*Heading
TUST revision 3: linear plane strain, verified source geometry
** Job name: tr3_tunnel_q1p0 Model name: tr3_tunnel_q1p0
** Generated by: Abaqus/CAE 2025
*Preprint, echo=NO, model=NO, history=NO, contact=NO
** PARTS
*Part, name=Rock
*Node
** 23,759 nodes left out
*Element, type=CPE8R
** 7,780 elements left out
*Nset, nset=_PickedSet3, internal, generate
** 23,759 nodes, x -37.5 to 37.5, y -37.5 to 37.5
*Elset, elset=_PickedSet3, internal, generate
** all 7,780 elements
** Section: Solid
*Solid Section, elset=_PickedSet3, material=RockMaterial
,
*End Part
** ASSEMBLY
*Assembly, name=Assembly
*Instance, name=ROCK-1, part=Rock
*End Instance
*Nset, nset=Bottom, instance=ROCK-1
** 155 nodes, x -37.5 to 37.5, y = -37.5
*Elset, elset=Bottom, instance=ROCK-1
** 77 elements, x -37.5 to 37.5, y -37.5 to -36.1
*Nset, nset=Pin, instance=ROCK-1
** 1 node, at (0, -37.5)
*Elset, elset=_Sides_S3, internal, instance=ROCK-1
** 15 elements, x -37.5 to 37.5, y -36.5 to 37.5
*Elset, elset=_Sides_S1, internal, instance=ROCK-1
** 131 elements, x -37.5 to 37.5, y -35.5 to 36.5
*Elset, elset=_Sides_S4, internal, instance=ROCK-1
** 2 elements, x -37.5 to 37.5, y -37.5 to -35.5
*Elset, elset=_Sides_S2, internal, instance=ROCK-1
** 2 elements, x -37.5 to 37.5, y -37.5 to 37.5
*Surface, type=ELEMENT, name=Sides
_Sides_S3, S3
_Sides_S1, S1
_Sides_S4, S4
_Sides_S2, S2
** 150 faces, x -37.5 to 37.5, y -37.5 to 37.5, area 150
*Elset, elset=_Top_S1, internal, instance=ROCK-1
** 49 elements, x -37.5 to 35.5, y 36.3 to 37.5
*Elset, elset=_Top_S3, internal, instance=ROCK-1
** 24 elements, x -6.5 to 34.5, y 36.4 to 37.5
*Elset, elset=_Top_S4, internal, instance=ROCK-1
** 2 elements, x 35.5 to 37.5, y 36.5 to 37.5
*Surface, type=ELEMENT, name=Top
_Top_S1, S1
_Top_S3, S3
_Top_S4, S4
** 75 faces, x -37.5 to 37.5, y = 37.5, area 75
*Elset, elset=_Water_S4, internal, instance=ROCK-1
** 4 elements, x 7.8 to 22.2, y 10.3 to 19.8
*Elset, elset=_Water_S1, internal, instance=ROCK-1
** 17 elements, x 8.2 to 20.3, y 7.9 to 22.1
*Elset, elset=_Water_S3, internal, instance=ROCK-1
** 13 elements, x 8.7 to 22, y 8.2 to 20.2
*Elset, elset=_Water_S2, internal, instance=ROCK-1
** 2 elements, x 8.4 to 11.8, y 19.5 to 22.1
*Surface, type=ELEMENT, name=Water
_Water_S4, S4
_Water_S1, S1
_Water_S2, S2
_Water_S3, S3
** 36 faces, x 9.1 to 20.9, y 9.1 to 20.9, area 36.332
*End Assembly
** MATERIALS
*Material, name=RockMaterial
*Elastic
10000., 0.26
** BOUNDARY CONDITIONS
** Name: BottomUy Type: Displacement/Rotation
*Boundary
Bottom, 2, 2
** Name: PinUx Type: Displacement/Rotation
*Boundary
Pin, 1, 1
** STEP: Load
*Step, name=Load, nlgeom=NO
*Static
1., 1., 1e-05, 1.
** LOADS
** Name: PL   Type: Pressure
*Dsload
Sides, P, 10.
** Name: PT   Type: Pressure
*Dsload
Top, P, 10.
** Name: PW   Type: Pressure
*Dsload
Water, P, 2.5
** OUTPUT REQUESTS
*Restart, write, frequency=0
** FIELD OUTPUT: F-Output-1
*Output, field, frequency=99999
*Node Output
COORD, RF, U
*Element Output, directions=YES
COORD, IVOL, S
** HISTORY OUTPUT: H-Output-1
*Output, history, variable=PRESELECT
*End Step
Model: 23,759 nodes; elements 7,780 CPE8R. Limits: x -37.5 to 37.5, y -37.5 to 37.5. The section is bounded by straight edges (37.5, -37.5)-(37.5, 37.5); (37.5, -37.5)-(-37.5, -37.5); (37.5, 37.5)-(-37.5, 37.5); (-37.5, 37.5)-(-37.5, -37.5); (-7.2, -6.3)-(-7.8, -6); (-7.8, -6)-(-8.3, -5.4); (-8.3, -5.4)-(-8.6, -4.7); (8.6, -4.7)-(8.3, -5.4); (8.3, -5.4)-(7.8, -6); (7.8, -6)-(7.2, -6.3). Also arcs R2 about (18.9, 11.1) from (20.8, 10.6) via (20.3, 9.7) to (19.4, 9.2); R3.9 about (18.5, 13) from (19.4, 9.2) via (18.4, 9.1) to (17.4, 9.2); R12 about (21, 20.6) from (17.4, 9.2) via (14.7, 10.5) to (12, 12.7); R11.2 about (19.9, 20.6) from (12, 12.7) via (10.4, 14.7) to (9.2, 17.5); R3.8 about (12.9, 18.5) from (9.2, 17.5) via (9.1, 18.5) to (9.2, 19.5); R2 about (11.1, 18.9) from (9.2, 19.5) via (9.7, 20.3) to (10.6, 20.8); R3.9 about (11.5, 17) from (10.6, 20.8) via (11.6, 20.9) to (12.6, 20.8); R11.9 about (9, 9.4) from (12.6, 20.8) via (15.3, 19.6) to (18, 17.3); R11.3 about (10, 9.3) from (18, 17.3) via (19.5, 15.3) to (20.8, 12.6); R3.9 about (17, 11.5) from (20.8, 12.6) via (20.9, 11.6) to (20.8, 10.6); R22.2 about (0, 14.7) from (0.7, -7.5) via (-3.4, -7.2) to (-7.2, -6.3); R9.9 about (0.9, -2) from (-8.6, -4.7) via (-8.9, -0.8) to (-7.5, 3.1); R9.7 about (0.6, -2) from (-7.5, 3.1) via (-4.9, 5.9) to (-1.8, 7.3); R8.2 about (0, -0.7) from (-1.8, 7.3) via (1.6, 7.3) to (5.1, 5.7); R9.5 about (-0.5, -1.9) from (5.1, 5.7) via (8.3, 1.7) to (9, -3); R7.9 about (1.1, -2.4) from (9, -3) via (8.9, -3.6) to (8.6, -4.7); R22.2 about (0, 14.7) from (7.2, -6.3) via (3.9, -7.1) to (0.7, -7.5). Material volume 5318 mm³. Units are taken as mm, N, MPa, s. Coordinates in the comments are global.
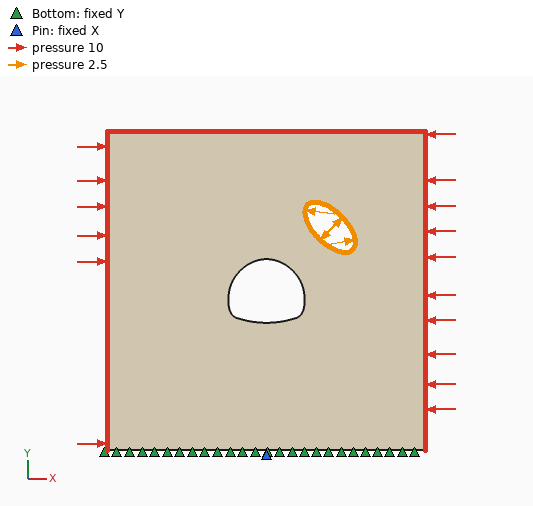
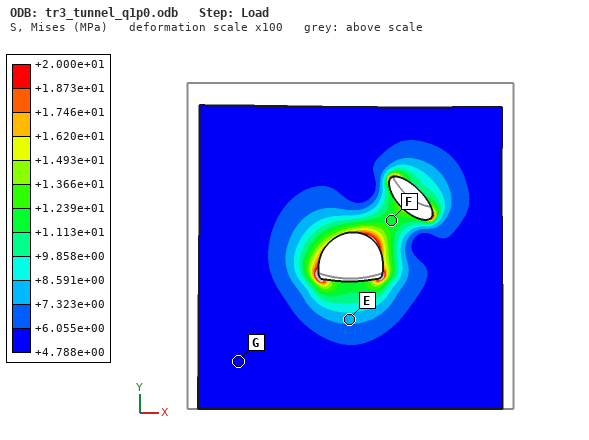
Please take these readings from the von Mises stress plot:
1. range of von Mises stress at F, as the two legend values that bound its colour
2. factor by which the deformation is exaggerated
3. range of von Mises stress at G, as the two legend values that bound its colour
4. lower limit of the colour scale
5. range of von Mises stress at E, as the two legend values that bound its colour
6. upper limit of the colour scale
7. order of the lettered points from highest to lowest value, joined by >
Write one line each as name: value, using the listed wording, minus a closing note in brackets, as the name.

range of von Mises stress at F, as the two legend values that bound its colour: +1.113e+01 to +1.239e+01 MPa
factor by which the deformation is exaggerated: 100
range of von Mises stress at G, as the two legend values that bound its colour: +4.788e+00 to +6.055e+00 MPa
lower limit of the colour scale: +4.788e+00 MPa
range of von Mises stress at E, as the two legend values that bound its colour: +7.323e+00 to +8.591e+00 MPa
upper limit of the colour scale: +2.000e+01 MPa
order of the lettered points from highest to lowest value, joined by >: F > E > G
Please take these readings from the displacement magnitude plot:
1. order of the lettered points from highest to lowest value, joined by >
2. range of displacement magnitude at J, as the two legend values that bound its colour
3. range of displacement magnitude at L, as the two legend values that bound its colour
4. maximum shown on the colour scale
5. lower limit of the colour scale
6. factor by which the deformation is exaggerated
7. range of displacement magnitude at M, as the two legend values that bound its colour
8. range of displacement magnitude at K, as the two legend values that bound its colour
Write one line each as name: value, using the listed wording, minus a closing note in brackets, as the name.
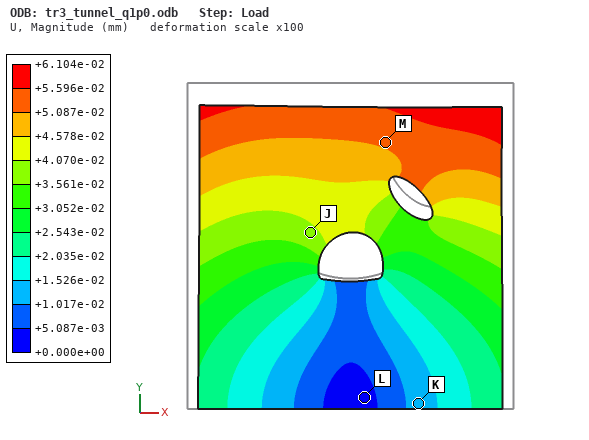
order of the lettered points from highest to lowest value, joined by >: M > J > K > L
range of displacement magnitude at J, as the two legend values that bound its colour: +3.561e-02 to +4.070e-02 mm
range of displacement magnitude at L, as the two legend values that bound its colour: +0.000e+00 to +5.087e-03 mm
maximum shown on the colour scale: +6.104e-02 mm
lower limit of the colour scale: +0.000e+00 mm
factor by which the deformation is exaggerated: 100
range of displacement magnitude at M, as the two legend values that bound its colour: +5.087e-02 to +5.596e-02 mm
range of displacement magnitude at K, as the two legend values that bound its colour: +1.017e-02 to +1.526e-02 mm
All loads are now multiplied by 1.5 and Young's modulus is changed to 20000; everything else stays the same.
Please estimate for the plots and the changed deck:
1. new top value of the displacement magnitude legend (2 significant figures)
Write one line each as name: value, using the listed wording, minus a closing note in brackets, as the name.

new top value of the displacement magnitude legend: 0.046 mm
